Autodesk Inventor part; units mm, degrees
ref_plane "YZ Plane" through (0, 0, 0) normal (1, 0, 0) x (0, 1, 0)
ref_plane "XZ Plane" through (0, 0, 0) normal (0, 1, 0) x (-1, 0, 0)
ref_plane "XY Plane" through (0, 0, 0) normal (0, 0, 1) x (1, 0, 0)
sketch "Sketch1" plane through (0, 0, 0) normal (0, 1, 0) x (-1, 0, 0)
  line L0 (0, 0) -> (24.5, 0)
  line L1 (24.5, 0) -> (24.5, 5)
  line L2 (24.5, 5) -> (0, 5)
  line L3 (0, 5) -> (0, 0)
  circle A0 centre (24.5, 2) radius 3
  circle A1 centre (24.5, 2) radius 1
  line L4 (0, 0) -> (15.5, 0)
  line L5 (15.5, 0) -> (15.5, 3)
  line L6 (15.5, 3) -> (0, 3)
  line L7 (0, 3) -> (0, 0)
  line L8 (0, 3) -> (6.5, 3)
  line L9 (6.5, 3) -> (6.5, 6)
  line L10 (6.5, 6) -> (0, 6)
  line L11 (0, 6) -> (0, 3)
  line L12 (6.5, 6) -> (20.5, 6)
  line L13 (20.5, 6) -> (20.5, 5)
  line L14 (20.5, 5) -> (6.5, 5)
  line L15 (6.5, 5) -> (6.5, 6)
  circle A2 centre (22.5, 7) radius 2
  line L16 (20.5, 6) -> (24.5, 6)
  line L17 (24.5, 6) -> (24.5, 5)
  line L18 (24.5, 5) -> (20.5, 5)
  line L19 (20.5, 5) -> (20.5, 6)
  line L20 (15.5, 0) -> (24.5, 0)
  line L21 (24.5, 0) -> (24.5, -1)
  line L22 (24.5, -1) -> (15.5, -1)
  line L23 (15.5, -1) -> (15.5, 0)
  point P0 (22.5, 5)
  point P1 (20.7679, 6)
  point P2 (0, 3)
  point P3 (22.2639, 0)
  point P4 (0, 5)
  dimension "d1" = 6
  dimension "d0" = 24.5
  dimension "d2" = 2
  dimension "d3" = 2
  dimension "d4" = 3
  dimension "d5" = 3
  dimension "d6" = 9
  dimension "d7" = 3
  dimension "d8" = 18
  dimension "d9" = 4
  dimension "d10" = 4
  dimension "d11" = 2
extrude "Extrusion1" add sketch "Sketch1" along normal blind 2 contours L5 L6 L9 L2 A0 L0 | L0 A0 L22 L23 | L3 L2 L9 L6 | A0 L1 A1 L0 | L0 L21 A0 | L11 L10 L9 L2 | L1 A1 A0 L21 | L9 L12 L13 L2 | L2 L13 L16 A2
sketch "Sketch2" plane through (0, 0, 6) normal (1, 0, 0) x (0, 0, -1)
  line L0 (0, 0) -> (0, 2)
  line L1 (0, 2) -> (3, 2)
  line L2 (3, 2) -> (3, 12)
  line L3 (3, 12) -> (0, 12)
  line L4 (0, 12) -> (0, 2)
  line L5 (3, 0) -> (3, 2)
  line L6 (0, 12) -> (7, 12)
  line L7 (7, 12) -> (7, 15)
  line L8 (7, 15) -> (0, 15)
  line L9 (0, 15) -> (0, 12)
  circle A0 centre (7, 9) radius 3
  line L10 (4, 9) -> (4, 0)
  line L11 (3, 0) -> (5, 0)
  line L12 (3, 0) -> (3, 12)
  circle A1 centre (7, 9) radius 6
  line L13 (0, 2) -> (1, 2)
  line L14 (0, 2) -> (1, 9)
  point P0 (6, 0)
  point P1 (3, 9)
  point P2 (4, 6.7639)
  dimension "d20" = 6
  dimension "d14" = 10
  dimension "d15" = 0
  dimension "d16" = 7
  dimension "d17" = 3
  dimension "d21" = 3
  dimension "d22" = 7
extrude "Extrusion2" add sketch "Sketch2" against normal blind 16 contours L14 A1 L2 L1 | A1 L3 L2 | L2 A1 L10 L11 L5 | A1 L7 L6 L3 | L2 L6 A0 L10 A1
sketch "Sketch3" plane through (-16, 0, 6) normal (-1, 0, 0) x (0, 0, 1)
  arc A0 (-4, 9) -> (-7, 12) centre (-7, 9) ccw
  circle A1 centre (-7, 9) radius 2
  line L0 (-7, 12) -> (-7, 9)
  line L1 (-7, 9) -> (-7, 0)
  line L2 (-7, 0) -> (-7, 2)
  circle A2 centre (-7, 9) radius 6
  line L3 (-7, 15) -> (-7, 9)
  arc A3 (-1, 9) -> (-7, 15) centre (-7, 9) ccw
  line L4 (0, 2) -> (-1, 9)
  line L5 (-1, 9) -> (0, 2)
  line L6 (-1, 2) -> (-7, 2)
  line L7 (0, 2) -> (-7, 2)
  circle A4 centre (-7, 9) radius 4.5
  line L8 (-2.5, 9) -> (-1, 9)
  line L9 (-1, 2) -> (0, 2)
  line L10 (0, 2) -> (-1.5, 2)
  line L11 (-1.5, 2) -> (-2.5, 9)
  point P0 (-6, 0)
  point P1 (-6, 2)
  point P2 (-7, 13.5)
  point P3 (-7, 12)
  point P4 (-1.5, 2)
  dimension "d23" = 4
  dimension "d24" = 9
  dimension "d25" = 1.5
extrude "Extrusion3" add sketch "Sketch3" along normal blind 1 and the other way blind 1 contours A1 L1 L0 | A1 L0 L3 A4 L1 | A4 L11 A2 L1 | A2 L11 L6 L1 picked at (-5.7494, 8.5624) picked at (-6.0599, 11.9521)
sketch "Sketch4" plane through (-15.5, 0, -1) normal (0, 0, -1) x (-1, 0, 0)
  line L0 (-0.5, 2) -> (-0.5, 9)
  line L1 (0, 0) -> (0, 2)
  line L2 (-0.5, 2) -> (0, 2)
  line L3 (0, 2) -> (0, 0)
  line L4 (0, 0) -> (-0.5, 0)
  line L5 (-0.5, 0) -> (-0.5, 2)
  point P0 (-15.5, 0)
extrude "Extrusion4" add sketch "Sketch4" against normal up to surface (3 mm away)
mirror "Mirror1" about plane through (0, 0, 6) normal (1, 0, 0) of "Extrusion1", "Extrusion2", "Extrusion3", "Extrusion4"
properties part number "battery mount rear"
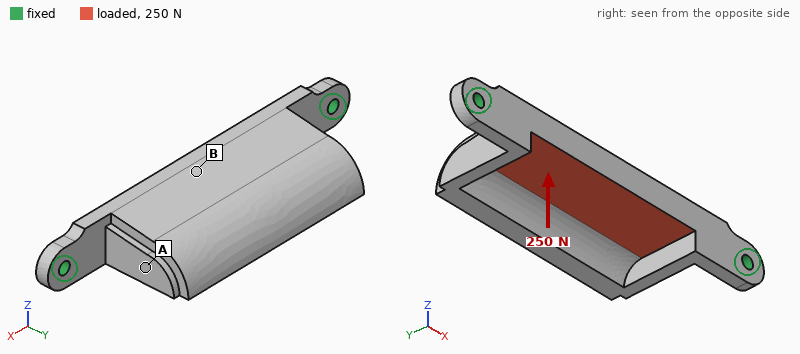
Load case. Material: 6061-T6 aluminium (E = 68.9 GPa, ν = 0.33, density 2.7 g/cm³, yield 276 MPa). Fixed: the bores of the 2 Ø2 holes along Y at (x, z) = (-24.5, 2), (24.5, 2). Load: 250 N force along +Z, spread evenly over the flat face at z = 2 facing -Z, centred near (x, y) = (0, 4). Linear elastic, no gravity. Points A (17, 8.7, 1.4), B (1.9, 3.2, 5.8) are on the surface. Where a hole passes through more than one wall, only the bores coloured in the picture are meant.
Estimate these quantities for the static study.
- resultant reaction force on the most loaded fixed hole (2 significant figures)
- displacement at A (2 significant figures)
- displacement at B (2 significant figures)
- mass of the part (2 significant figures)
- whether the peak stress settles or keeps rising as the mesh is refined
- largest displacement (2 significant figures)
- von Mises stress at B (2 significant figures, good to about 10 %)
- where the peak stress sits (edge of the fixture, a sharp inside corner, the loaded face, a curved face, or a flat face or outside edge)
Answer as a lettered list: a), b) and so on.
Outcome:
a) 210 N
b) 0.081 mm
c) 0.063 mm
d) 5.8 g
e) keeps rising
f) 0.15 mm
g) 31 MPa
h) edge of the fixture
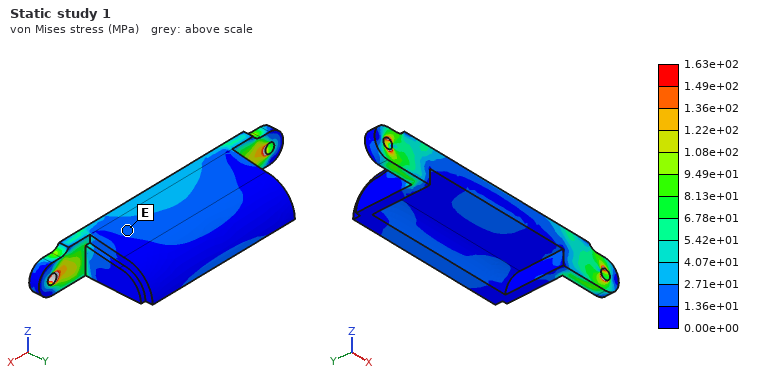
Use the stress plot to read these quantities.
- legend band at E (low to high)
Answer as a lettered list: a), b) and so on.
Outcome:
a) 1.36e+01 to 2.71e+01 MPa
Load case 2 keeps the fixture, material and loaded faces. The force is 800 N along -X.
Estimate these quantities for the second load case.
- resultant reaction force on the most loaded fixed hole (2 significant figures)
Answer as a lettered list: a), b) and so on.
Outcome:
a) 410 N
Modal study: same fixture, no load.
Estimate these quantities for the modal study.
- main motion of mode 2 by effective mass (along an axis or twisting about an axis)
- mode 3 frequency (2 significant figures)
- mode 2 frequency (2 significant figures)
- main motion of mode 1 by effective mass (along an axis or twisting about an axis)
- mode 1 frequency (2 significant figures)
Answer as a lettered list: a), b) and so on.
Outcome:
a) along Y
b) 9600 Hz
c) 6600 Hz
d) along Z
e) 2700 Hz
